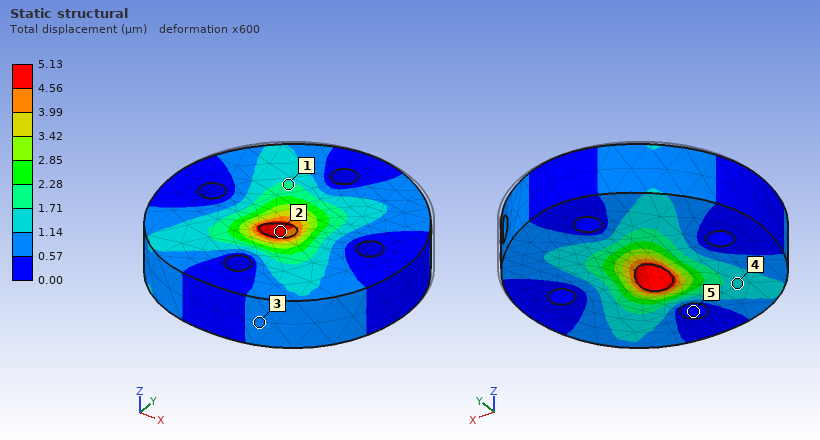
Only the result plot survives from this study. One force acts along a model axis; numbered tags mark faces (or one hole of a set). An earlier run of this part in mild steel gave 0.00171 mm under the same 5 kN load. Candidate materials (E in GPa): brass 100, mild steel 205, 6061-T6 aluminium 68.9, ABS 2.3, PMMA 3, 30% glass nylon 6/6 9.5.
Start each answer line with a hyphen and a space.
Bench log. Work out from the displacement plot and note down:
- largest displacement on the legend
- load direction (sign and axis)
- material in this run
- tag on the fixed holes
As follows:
- 5.13 µm
- -Y
- 6061-T6 aluminium
- 5
